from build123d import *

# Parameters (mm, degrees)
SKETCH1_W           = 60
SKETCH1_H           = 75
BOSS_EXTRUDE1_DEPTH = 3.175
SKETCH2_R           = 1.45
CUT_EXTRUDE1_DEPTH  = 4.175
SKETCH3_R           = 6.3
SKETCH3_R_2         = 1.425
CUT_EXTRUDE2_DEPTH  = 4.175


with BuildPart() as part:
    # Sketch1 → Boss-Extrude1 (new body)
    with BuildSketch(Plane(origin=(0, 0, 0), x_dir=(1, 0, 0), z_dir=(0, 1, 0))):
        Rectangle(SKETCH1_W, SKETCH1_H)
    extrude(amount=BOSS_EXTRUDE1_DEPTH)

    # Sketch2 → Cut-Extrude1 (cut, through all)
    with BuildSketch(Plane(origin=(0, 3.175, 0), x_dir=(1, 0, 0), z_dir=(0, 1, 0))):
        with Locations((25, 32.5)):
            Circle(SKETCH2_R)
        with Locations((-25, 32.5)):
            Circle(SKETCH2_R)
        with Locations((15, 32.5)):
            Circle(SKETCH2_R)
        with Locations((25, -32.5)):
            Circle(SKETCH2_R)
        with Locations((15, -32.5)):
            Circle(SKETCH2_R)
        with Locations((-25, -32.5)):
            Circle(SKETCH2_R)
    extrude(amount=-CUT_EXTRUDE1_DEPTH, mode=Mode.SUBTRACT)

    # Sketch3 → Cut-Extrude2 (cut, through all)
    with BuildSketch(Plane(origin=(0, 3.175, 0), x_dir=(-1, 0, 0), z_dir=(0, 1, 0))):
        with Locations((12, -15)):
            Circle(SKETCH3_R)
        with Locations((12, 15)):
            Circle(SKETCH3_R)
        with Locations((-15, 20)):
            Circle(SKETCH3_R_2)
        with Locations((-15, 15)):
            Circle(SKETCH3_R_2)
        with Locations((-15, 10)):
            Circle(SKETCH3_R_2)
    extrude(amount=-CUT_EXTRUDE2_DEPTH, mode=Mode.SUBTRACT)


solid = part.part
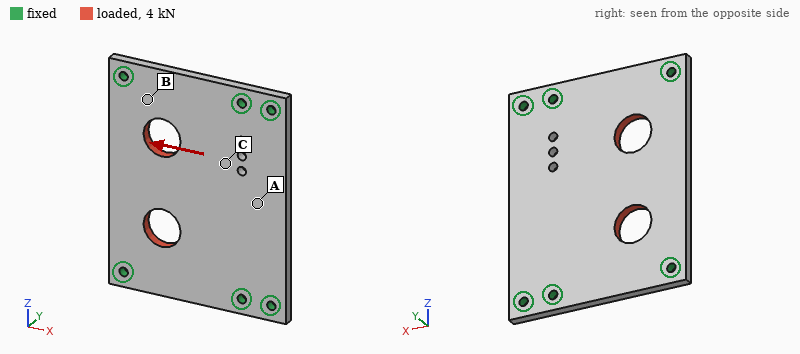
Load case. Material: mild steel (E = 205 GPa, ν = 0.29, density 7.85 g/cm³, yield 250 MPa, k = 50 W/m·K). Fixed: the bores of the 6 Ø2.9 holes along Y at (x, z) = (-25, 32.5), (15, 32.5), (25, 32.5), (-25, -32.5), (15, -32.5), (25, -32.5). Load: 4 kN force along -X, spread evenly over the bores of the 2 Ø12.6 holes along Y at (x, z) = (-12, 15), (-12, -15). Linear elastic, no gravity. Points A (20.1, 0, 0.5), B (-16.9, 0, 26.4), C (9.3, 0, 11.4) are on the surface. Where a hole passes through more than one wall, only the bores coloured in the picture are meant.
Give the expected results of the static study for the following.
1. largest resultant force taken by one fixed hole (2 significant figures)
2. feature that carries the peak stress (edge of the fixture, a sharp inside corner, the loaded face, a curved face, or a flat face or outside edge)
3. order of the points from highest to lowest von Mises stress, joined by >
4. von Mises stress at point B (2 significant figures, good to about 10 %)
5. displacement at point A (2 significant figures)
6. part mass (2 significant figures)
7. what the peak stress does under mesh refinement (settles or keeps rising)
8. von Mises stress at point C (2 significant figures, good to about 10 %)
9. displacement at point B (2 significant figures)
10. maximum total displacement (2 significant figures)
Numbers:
960 N
edge of the fixture
B > C > A
24 MPa
3.5 µm
100 g
keeps rising
14 MPa
1.8 µm
5.5 µm
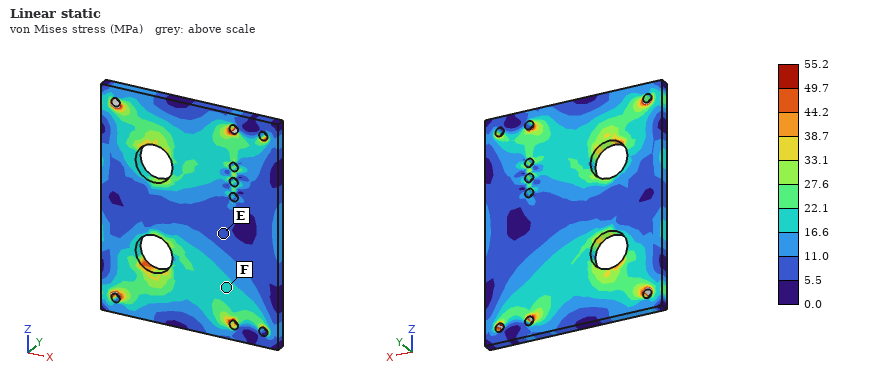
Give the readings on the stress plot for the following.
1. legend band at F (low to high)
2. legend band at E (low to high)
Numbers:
16.6 to 22.1 MPa
5.5 to 11.0 MPa
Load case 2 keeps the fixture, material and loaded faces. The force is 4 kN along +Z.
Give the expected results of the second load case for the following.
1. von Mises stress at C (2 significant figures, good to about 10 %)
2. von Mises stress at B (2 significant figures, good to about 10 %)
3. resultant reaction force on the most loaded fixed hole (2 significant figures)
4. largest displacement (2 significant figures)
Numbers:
10 MPa
19 MPa
1.2 kN
3.7 µm
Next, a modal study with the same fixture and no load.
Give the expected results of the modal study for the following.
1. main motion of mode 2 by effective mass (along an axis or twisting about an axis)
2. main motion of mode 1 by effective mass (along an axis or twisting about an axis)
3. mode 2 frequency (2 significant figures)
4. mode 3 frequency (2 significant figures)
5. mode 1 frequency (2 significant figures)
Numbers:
twisting about Z
along Y
4700 Hz
7200 Hz
3400 Hz
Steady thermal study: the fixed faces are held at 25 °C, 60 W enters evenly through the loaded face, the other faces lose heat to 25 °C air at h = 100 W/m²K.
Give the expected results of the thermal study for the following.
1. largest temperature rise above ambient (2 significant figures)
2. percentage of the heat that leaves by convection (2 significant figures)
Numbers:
84 K
47 %
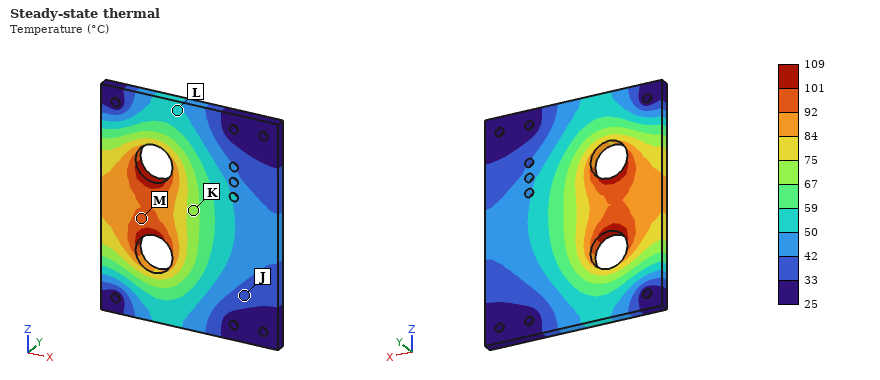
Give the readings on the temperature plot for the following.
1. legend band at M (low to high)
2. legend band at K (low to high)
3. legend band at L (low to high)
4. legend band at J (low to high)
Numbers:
92 to 101 °C
67 to 75 °C
50 to 59 °C
33 to 42 °C
